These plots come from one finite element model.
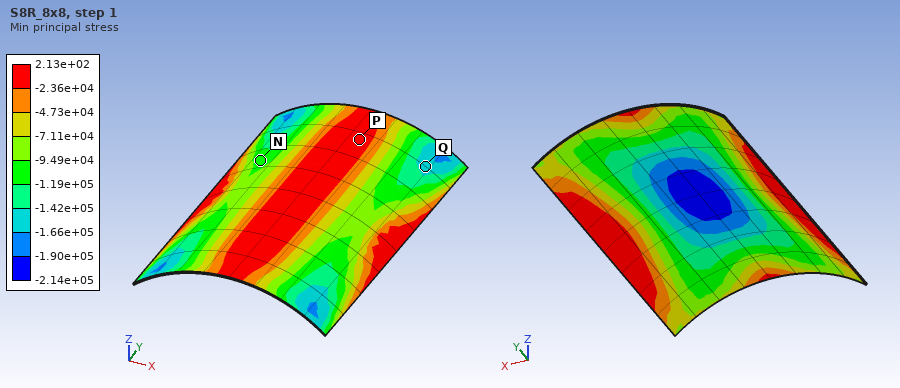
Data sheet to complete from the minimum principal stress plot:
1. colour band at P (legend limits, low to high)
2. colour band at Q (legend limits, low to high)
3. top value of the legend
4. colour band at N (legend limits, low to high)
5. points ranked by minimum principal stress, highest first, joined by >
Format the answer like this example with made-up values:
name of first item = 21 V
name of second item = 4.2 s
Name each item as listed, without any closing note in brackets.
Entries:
colour band at P = -2.36e+04 to 2.13e+02
colour band at Q = -1.66e+05 to -1.42e+05
top value of the legend = 2.13e+02
colour band at N = -1.19e+05 to -9.49e+04
points ranked by minimum principal stress, highest first, joined by > = P > N > Q
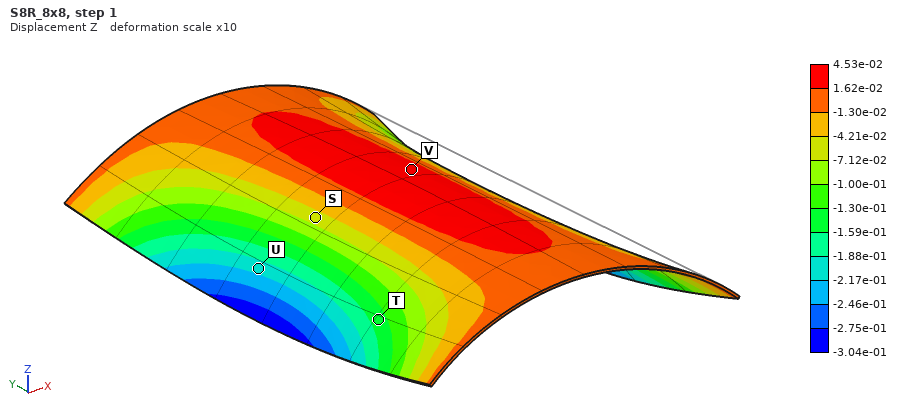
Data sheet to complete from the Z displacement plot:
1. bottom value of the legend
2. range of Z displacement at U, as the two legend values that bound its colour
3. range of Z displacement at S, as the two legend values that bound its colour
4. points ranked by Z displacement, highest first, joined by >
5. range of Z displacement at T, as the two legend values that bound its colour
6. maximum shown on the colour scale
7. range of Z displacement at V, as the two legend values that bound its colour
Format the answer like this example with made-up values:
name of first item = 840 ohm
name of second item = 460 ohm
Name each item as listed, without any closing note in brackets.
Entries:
bottom value of the legend = -3.04e-01
range of Z displacement at U, as the two legend values that bound its colour = -2.17e-01 to -1.88e-01
range of Z displacement at S, as the two legend values that bound its colour = -7.12e-02 to -4.21e-02
points ranked by Z displacement, highest first, joined by > = V > S > T > U
range of Z displacement at T, as the two legend values that bound its colour = -1.59e-01 to -1.30e-01
maximum shown on the colour scale = 4.53e-02
range of Z displacement at V, as the two legend values that bound its colour = 1.62e-02 to 4.53e-02
